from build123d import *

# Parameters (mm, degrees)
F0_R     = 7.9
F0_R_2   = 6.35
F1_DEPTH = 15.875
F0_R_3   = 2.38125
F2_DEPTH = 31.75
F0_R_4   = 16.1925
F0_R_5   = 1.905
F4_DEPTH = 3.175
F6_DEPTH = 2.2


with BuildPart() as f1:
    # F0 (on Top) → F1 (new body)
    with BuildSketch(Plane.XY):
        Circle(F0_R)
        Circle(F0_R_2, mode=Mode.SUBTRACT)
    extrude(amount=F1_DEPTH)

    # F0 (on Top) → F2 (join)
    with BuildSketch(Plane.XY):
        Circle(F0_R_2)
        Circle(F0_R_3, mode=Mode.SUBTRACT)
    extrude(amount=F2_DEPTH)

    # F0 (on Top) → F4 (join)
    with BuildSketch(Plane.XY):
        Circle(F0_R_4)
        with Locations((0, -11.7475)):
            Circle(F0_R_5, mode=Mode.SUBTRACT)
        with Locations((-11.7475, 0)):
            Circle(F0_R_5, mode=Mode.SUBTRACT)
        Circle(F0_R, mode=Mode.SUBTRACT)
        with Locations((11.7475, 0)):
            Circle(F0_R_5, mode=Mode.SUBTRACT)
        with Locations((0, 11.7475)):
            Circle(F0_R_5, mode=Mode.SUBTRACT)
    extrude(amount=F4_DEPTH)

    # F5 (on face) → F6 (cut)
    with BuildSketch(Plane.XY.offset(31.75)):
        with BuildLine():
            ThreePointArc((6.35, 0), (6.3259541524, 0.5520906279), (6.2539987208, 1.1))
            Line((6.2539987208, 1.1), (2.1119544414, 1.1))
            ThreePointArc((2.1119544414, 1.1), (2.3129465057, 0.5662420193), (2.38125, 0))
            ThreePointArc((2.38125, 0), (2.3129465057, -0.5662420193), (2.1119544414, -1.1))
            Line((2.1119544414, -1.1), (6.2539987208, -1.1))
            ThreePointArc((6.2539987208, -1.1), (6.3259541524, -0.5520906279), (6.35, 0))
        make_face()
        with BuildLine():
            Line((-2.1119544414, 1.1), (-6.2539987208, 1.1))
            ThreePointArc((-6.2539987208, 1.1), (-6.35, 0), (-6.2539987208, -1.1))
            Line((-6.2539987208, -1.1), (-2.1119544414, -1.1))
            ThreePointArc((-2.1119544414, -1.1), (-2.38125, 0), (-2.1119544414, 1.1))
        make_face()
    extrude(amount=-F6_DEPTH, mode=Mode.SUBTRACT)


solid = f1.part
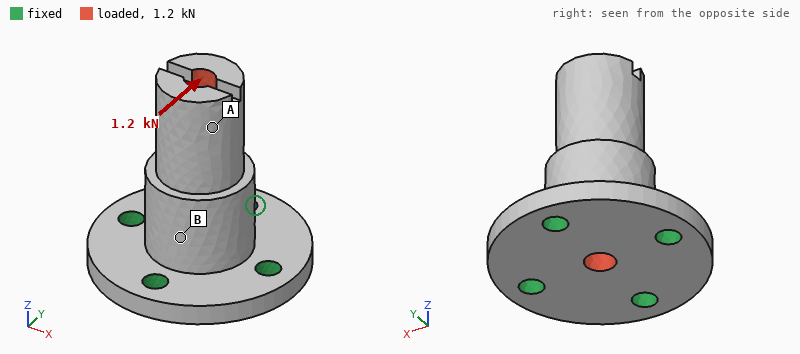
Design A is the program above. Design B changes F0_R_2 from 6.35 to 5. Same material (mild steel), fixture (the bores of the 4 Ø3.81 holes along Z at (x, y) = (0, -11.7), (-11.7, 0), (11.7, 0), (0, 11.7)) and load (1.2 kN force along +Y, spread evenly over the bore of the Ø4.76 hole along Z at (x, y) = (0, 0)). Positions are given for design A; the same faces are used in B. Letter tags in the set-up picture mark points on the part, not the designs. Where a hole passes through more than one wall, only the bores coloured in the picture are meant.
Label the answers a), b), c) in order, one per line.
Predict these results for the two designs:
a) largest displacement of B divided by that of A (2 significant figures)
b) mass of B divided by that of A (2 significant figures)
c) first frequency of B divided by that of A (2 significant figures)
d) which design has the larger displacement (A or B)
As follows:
a) 1.2
b) 0.88
c) 1.2
d) B
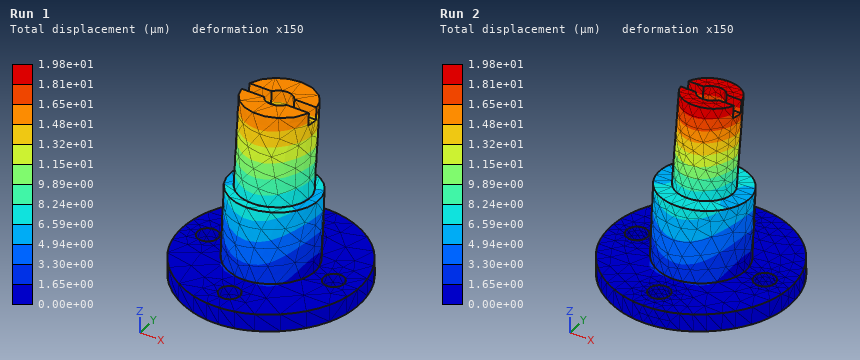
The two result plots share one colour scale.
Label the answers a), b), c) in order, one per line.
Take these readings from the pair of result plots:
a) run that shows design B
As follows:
a) Run 2
